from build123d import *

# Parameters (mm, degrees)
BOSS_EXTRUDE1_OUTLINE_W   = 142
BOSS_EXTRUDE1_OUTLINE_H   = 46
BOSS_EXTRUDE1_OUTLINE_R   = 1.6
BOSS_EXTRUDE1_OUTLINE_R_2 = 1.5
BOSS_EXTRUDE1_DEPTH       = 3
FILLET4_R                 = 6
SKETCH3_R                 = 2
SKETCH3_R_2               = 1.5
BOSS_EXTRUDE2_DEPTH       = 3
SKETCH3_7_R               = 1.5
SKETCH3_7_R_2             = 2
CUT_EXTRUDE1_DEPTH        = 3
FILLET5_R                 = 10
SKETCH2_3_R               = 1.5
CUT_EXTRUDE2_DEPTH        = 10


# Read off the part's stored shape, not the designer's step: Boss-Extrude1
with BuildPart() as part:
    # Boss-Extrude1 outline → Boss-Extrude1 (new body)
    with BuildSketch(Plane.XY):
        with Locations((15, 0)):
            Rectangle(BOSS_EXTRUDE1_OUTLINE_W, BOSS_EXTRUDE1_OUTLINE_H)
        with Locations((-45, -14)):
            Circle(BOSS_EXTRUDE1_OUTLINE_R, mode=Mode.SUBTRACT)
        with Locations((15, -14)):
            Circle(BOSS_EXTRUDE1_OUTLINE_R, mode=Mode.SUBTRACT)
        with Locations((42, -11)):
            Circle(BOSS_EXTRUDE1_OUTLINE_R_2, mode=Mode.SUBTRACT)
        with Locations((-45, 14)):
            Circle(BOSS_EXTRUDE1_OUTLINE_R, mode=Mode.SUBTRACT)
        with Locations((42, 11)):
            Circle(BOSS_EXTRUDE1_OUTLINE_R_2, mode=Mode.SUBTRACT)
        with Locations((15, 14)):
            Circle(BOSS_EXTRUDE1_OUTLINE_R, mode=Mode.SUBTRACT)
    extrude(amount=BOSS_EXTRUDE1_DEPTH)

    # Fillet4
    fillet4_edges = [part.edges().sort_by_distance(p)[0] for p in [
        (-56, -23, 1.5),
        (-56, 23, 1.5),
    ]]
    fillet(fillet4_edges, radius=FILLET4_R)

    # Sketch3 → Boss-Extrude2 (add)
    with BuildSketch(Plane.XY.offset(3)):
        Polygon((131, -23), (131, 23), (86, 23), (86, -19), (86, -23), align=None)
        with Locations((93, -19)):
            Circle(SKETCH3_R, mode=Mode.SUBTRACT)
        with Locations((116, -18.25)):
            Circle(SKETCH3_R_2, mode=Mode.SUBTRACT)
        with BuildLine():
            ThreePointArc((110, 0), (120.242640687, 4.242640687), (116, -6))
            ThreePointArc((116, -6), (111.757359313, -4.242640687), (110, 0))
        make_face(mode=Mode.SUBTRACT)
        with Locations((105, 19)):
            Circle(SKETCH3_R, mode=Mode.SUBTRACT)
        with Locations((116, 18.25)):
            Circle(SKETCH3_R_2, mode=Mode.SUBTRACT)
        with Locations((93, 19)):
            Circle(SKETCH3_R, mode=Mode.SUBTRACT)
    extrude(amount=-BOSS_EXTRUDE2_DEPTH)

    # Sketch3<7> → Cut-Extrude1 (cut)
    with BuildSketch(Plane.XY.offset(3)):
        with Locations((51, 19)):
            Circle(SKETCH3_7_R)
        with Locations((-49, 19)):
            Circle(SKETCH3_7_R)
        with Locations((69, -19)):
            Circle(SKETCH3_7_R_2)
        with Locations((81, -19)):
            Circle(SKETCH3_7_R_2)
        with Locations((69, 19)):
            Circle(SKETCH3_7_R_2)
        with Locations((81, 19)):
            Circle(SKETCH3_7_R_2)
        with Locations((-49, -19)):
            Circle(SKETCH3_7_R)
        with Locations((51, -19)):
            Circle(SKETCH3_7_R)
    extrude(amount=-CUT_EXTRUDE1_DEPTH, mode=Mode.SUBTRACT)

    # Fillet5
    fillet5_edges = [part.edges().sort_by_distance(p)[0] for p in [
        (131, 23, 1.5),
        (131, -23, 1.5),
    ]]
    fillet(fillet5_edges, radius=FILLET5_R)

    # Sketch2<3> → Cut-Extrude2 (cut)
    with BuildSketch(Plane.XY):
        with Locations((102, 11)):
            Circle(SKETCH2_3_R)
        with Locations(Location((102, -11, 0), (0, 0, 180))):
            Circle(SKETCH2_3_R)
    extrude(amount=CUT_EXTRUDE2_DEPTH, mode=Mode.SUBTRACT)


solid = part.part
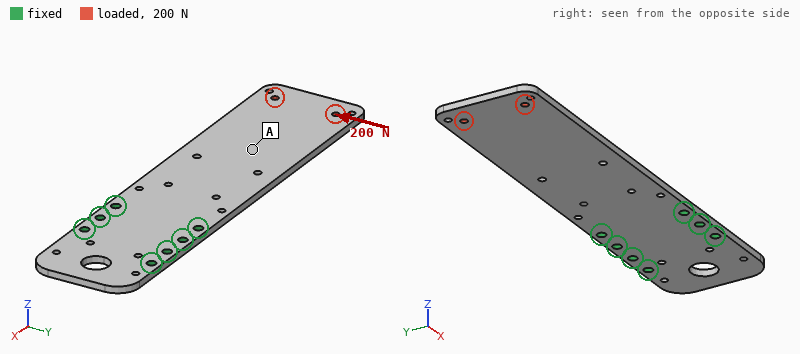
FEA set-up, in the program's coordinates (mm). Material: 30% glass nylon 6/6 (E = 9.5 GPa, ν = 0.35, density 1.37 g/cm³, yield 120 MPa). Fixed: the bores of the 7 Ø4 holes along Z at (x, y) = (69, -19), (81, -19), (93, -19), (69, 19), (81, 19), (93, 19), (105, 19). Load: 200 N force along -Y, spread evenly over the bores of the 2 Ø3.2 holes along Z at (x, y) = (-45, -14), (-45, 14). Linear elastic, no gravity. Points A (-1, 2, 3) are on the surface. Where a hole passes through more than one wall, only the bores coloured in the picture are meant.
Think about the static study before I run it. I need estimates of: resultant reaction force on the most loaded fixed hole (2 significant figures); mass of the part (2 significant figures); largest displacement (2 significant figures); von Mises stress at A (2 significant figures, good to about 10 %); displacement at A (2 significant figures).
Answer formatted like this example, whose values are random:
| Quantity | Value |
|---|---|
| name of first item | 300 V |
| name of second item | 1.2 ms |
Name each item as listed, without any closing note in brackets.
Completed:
| Quantity | Value |
|---|---|
| resultant reaction force on the most loaded fixed hole | 540 N |
| mass of the part | 34 g |
| largest displacement | 0.58 mm |
| von Mises stress at A | 3.7 MPa |
| displacement at A | 0.24 mm |
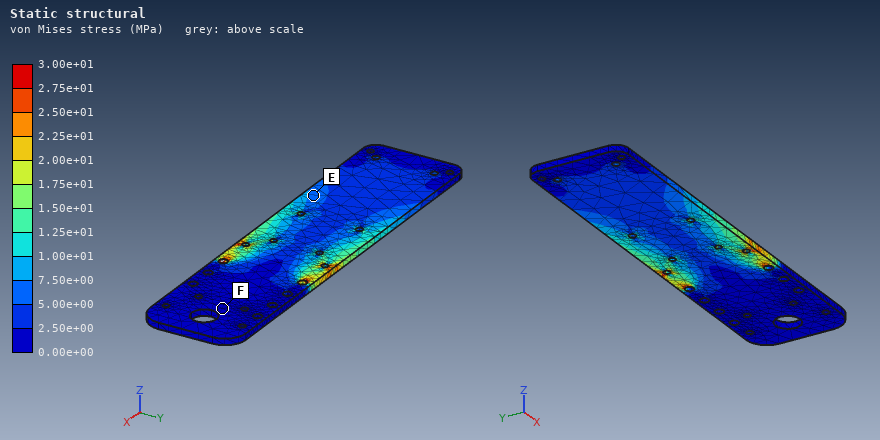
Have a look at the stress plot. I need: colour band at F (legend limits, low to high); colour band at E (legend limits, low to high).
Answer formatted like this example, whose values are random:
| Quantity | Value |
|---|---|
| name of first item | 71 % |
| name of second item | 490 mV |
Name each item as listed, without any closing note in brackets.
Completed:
| Quantity | Value |
|---|---|
| colour band at F | 0.00e+00 to 2.50e+00 MPa |
| colour band at E | 5.00e+00 to 7.50e+00 MPa |
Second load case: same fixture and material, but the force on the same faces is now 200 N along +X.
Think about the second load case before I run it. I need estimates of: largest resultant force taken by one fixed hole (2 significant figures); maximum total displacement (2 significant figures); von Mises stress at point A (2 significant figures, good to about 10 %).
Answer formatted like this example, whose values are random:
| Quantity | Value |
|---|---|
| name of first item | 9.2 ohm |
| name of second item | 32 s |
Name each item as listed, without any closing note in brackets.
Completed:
| Quantity | Value |
|---|---|
| largest resultant force taken by one fixed hole | 70 N |
| maximum total displacement | 21 µm |
| von Mises stress at point A | 1.5 MPa |
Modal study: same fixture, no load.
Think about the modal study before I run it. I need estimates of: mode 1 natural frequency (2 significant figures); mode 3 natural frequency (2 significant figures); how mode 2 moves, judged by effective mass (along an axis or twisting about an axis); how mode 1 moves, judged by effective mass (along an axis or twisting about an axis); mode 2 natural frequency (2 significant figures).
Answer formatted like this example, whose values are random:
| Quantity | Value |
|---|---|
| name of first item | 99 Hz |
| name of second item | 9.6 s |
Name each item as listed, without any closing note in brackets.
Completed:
| Quantity | Value |
|---|---|
| mode 1 natural frequency | 81 Hz |
| mode 3 natural frequency | 510 Hz |
| how mode 2 moves, judged by effective mass | twisting about X |
| how mode 1 moves, judged by effective mass | along Z |
| mode 2 natural frequency | 460 Hz |
